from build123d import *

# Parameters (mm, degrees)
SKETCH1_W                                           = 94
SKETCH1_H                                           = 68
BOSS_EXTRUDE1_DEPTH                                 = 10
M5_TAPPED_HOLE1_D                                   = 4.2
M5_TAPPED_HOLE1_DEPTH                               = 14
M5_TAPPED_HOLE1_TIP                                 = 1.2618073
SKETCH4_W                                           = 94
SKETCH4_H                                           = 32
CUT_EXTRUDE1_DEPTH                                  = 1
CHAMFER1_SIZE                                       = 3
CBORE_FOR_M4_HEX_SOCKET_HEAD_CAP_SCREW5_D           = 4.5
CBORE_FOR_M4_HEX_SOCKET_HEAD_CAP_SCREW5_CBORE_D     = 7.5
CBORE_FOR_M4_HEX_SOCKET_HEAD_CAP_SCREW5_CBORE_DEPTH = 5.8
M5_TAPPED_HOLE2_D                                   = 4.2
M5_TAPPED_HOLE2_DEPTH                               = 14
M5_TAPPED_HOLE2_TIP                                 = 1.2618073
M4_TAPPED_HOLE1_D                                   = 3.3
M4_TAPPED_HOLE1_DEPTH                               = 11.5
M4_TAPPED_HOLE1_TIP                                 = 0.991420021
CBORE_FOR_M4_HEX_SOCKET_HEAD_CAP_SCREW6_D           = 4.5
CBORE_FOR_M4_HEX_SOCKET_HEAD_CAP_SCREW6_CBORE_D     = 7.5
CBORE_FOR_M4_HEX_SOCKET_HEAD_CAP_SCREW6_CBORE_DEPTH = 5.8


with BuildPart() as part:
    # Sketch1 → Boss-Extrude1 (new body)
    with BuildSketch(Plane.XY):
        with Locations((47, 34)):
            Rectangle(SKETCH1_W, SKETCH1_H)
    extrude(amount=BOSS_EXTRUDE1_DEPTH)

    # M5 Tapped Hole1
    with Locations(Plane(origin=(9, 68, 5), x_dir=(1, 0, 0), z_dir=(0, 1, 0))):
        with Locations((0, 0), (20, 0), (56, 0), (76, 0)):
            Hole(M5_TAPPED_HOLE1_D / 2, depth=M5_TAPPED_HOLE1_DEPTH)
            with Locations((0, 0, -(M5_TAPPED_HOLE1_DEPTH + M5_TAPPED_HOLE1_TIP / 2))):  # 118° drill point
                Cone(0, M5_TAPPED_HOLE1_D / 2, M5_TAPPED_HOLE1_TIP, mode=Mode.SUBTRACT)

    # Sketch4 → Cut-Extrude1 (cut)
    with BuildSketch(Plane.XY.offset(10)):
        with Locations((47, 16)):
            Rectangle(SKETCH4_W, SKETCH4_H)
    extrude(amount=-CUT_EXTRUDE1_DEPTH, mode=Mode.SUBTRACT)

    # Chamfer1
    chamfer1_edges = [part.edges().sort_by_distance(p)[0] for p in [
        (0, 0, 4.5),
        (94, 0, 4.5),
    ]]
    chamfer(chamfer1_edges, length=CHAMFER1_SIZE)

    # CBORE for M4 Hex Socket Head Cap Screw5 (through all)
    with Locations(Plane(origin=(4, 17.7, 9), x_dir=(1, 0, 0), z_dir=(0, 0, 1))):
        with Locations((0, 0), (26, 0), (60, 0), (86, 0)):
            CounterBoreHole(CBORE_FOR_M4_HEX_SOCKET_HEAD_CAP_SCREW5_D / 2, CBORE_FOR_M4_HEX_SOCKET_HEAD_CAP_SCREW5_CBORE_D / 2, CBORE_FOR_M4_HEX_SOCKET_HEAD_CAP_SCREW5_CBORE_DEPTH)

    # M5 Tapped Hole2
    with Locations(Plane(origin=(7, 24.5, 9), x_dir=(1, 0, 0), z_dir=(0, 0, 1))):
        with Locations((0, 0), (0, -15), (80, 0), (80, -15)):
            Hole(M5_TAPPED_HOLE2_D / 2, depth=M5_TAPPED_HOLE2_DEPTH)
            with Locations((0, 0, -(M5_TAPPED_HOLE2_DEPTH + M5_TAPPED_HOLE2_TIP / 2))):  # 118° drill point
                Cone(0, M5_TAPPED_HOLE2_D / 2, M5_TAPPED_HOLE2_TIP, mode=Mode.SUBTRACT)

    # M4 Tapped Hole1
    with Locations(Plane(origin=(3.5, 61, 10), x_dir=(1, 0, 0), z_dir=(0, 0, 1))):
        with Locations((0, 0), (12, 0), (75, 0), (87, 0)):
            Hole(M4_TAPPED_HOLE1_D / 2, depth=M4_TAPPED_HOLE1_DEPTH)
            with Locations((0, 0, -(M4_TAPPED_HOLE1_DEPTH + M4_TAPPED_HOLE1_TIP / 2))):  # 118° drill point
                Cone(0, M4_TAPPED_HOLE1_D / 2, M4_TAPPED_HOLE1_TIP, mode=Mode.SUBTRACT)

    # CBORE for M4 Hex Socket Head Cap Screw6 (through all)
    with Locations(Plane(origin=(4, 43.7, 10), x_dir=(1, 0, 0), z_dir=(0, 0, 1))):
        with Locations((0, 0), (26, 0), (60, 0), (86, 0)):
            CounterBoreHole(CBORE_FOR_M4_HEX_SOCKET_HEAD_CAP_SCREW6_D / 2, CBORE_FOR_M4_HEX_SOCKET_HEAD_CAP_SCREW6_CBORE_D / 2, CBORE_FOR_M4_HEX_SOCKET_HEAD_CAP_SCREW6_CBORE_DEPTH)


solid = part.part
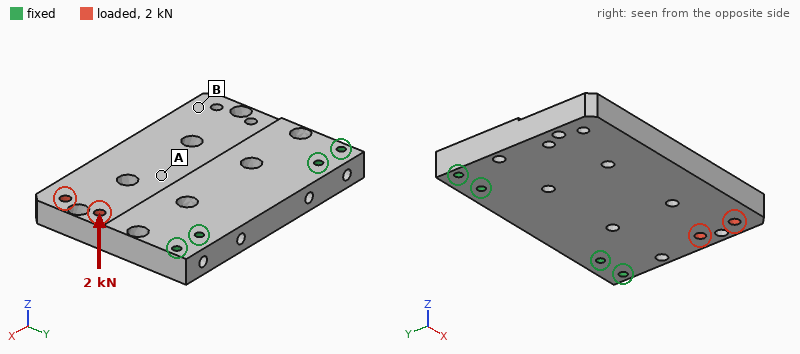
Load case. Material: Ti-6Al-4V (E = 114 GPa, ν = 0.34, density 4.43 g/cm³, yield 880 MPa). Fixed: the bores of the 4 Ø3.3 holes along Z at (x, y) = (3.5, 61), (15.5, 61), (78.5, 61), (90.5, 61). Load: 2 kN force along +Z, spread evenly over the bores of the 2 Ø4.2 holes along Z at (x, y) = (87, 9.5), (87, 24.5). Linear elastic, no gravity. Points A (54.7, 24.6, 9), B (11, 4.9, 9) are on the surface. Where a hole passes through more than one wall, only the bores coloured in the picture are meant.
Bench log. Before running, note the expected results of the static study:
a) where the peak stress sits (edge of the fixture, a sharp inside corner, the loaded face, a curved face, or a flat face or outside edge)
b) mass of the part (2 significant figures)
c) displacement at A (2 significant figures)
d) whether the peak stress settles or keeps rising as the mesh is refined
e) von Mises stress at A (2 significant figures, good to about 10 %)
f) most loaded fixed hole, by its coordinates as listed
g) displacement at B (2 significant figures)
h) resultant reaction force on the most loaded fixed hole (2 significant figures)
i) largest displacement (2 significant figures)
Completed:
edge of the fixture
250 g
0.092 mm
keeps rising
32 MPa
(78.5, 61)
0.082 mm
1.3 kN
0.28 mm
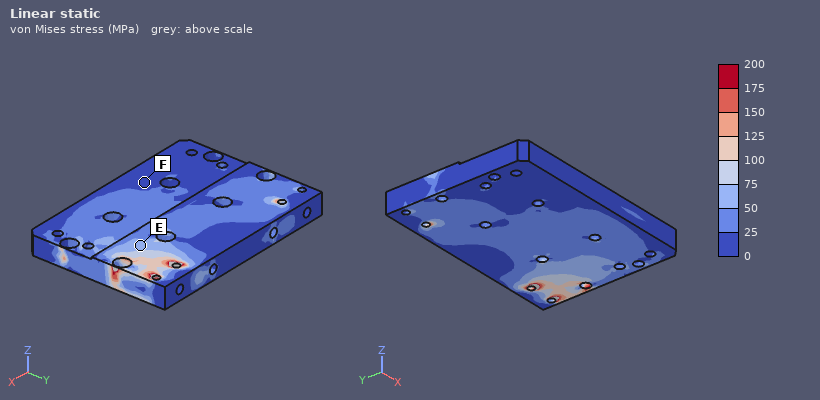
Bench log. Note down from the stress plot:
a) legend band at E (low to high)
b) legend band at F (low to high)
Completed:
50 to 75 MPa
0 to 25 MPa
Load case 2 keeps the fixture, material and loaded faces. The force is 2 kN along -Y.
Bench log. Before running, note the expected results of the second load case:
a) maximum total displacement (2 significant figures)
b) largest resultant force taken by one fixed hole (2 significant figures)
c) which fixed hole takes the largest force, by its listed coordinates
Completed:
7.4 µm
1.3 kN
(78.5, 61)
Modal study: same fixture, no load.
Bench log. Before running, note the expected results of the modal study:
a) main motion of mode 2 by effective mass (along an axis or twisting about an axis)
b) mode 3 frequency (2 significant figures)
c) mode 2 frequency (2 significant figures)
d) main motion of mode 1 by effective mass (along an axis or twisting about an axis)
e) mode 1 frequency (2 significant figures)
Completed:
twisting about Y
7400 Hz
3600 Hz
along Z
1800 Hz
